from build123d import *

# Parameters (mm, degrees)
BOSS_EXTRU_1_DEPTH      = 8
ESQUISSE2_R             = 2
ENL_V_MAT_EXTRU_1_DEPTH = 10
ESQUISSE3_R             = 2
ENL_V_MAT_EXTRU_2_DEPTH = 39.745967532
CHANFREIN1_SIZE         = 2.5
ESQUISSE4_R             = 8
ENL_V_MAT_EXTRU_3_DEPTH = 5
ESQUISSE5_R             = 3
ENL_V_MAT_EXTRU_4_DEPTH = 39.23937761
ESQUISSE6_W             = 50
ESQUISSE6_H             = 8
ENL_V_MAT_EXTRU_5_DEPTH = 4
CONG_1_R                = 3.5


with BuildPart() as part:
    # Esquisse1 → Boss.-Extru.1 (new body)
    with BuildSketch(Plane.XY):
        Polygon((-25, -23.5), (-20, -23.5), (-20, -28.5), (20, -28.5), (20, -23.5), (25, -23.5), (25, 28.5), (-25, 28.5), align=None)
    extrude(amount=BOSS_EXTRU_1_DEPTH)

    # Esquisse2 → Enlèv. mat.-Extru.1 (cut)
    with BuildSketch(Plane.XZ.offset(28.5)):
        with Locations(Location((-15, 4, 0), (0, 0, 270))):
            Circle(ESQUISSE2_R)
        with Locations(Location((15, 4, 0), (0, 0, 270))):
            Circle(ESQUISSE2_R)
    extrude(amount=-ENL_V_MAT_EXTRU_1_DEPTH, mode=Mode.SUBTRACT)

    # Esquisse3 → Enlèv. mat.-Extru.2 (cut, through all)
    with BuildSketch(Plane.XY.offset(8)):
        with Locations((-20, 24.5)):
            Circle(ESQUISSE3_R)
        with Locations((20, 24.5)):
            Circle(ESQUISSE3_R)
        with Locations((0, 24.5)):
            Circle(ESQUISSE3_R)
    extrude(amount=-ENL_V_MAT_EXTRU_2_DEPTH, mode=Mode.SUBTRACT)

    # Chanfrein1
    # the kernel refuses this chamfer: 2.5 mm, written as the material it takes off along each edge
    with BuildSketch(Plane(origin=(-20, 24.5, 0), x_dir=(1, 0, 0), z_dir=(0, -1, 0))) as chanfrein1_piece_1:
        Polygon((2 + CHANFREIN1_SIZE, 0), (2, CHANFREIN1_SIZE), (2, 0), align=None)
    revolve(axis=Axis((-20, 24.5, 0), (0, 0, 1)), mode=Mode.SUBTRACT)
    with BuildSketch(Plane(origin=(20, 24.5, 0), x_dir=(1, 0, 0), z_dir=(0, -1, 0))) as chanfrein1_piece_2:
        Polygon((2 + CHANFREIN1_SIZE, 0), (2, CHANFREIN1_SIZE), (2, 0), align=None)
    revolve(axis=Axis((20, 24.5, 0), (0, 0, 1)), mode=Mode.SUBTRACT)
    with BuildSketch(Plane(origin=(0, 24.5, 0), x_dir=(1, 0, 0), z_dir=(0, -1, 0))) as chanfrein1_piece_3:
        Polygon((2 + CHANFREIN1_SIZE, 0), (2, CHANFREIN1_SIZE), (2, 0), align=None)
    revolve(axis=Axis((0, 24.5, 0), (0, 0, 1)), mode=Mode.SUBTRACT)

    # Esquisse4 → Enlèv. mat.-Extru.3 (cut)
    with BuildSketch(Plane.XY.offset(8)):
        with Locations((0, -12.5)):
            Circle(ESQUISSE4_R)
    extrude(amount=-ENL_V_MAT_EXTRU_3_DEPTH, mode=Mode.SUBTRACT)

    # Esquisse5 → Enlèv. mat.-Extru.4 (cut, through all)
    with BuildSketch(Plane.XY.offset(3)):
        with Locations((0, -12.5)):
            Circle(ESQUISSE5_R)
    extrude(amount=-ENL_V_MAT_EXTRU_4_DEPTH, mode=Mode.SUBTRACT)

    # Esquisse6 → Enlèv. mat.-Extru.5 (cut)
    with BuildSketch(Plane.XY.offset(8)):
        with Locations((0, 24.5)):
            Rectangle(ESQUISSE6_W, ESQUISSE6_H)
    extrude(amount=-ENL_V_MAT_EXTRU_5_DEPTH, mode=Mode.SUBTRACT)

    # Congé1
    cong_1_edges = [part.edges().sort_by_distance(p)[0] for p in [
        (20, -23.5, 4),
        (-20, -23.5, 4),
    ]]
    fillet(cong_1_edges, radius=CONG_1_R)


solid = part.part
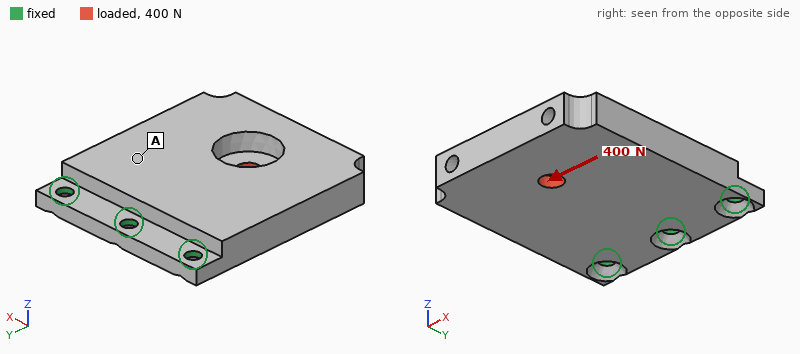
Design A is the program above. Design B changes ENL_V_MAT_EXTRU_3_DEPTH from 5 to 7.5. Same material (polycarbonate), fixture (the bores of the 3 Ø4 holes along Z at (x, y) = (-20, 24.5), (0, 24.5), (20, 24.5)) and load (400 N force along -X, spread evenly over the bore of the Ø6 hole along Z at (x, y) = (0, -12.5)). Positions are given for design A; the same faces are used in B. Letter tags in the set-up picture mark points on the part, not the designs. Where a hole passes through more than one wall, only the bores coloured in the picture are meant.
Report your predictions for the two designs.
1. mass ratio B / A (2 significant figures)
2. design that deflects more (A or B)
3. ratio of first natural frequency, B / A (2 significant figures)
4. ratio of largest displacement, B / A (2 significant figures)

0.98
B
1.0
1.3
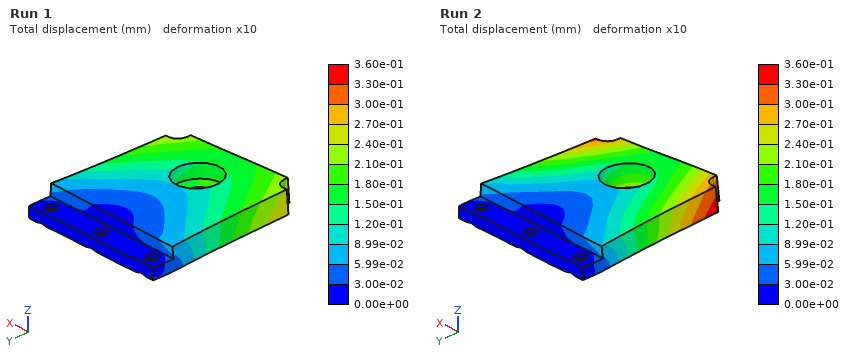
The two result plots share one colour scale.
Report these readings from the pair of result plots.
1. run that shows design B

Run 2
